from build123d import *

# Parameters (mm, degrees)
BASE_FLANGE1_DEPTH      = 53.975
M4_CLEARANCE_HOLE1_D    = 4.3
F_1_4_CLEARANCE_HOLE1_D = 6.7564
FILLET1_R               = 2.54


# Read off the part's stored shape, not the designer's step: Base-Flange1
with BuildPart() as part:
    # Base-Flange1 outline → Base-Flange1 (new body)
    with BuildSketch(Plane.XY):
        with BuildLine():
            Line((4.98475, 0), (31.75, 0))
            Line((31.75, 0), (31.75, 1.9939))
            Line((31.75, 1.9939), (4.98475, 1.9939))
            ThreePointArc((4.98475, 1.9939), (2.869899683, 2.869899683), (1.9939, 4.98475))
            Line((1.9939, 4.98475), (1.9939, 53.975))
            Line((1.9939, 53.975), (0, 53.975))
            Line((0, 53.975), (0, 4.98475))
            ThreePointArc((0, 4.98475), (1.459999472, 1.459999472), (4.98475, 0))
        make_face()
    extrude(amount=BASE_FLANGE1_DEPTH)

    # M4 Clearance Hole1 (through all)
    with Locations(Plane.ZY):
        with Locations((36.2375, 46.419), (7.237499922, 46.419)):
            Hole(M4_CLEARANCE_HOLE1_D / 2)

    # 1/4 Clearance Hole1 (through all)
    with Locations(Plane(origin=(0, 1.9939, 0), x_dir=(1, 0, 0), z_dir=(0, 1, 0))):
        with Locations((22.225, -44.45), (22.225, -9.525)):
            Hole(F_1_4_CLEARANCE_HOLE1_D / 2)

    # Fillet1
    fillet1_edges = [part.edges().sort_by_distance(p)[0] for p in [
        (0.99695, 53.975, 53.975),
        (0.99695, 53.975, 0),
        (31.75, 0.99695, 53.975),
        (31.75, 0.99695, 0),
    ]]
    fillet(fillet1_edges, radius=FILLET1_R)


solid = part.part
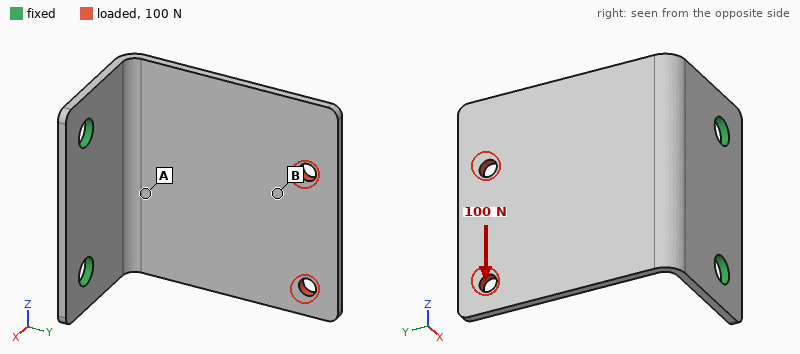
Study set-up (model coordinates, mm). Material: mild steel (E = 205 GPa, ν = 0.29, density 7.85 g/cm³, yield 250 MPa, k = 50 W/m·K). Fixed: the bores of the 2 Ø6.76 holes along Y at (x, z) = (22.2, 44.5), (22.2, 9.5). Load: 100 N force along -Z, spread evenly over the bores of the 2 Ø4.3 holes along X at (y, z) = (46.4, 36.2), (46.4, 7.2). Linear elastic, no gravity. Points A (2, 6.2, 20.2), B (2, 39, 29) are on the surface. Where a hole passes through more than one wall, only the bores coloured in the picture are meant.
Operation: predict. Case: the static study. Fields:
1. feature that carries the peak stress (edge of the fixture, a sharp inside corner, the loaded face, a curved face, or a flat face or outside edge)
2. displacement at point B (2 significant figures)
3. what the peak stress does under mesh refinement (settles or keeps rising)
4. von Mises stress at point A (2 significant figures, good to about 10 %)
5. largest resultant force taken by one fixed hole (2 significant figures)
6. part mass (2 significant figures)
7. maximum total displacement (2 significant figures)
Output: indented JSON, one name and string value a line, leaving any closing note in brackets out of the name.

{
  "feature that carries the peak stress": "edge of the fixture",
  "displacement at point B": "0.087 mm",
  "what the peak stress does under mesh refinement": "keeps rising",
  "von Mises stress at point A": "30 MPa",
  "largest resultant force taken by one fixed hole": "140 N",
  "part mass": "68 g",
  "maximum total displacement": "0.14 mm"
}
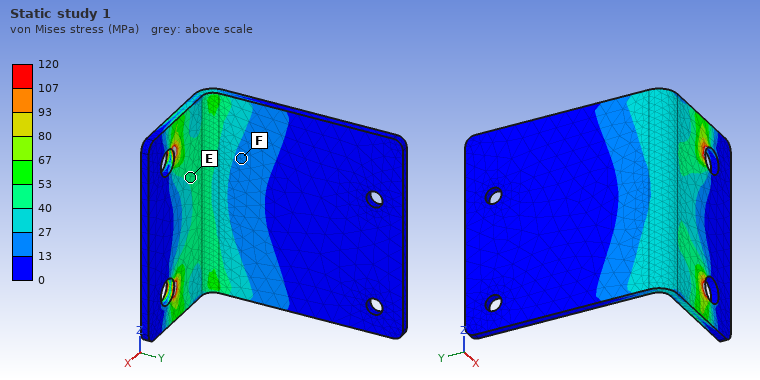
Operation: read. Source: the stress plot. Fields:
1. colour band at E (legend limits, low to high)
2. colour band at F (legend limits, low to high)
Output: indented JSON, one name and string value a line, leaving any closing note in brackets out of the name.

{
  "colour band at E": "40 to 53 MPa",
  "colour band at F": "13 to 27 MPa"
}
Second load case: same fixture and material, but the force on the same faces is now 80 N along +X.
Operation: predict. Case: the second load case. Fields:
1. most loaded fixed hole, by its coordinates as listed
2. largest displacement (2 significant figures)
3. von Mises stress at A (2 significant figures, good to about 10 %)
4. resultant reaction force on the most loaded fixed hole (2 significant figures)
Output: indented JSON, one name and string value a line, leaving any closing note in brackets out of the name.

{
  "most loaded fixed hole, by its coordinates as listed": "(22.2, 9.5)",
  "largest displacement": "0.89 mm",
  "von Mises stress at A": "87 MPa",
  "resultant reaction force on the most loaded fixed hole": "55 N"
}
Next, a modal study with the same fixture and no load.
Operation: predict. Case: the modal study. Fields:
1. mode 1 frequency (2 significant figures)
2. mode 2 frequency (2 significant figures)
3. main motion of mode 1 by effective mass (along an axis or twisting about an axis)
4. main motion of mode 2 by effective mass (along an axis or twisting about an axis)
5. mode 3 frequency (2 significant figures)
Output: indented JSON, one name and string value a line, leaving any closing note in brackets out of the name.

{
  "mode 1 frequency": "390 Hz",
  "mode 2 frequency": "930 Hz",
  "main motion of mode 1 by effective mass": "along X",
  "main motion of mode 2 by effective mass": "along Z",
  "mode 3 frequency": "1500 Hz"
}
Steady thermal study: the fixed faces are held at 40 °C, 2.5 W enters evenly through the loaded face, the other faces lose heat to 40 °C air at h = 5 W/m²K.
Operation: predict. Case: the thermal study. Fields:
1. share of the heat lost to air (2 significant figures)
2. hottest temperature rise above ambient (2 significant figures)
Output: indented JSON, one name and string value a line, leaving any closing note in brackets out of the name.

{
  "share of the heat lost to air": "23 %",
  "hottest temperature rise above ambient": "30 K"
}
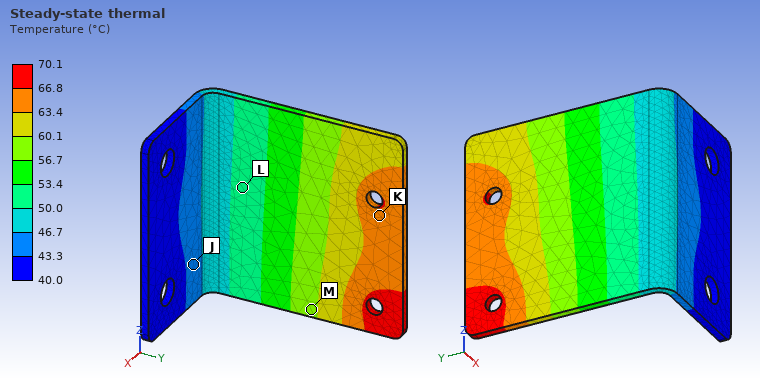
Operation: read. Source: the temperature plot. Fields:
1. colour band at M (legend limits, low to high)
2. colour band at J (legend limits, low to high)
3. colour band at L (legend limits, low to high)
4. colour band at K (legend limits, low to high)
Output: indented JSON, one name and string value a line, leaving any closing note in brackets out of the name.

{
  "colour band at M": "56.7 to 60.1 °C",
  "colour band at J": "43.3 to 46.7 °C",
  "colour band at L": "50.0 to 53.4 °C",
  "colour band at K": "63.4 to 66.8 °C"
}
